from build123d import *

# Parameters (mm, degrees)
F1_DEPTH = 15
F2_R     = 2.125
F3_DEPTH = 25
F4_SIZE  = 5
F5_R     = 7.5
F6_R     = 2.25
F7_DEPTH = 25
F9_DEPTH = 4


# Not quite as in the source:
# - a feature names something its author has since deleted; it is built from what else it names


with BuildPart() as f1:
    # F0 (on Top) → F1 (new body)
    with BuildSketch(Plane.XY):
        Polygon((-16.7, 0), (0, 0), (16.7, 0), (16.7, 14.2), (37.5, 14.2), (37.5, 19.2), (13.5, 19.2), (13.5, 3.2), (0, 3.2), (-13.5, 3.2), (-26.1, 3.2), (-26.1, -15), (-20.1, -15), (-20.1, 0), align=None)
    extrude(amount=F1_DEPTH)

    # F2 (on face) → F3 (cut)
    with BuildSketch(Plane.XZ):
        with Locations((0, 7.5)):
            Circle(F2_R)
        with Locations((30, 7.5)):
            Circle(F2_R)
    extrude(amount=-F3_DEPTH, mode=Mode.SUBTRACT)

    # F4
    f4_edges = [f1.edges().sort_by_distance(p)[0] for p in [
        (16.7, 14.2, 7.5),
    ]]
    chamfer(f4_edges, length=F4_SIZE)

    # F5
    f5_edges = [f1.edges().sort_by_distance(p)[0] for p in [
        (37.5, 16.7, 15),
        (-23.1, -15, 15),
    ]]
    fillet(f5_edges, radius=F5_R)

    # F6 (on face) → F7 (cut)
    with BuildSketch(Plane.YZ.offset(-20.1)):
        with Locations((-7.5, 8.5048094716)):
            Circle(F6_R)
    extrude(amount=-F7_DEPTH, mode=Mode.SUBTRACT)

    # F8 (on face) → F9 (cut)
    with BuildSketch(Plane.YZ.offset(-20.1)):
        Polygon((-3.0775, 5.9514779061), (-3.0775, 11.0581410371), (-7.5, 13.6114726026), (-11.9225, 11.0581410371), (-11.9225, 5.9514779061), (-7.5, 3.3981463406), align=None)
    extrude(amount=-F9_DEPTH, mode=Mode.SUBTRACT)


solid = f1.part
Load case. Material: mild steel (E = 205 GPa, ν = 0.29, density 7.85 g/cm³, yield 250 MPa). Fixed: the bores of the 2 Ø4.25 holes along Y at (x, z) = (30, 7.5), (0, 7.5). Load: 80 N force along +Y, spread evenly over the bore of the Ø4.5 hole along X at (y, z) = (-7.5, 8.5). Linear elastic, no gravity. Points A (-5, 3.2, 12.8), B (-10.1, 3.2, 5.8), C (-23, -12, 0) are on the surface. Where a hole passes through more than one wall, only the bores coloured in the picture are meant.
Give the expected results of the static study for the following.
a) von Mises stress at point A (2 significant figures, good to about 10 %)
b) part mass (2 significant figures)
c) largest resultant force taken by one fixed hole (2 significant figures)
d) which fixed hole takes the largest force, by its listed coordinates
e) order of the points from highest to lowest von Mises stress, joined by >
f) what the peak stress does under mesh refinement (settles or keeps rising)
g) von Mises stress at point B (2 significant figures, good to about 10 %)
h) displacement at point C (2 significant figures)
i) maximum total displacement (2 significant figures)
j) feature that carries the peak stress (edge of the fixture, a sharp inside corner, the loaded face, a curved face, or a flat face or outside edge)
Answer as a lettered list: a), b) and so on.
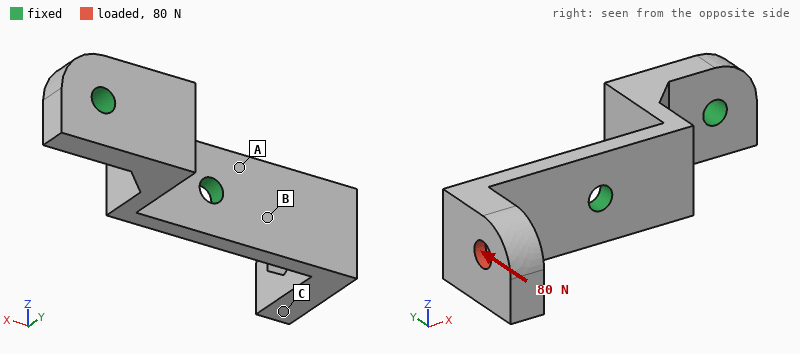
a) 56 MPa
b) 42 g
c) 93 N
d) (0, 7.5)
e) A > B > C
f) keeps rising
g) 43 MPa
h) 53 µm
i) 66 µm
j) edge of the fixture
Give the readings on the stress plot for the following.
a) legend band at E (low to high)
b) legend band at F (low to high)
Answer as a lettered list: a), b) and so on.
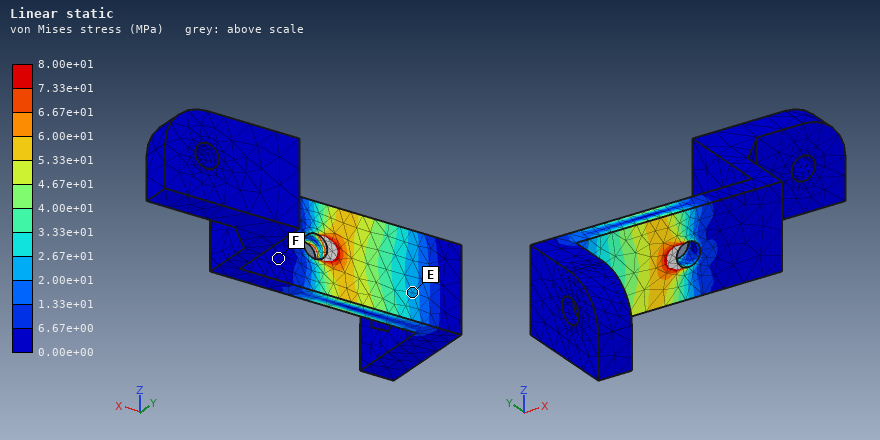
a) 2.00e+01 to 2.67e+01 MPa
b) 0.00e+00 to 6.67e+00 MPa
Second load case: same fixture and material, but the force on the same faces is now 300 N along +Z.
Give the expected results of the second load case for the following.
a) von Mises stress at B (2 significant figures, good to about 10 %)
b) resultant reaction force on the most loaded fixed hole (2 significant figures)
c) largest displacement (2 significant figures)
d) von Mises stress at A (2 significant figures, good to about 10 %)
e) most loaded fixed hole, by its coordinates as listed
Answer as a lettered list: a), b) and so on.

a) 82 MPa
b) 370 N
c) 95 µm
d) 86 MPa
e) (0, 7.5)
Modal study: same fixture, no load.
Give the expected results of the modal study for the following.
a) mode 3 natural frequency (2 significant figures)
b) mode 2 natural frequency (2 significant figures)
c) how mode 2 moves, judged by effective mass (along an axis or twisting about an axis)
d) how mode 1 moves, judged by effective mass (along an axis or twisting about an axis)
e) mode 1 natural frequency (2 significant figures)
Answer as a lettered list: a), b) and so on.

a) 7800 Hz
b) 3700 Hz
c) along Z
d) along Y
e) 2000 Hz
